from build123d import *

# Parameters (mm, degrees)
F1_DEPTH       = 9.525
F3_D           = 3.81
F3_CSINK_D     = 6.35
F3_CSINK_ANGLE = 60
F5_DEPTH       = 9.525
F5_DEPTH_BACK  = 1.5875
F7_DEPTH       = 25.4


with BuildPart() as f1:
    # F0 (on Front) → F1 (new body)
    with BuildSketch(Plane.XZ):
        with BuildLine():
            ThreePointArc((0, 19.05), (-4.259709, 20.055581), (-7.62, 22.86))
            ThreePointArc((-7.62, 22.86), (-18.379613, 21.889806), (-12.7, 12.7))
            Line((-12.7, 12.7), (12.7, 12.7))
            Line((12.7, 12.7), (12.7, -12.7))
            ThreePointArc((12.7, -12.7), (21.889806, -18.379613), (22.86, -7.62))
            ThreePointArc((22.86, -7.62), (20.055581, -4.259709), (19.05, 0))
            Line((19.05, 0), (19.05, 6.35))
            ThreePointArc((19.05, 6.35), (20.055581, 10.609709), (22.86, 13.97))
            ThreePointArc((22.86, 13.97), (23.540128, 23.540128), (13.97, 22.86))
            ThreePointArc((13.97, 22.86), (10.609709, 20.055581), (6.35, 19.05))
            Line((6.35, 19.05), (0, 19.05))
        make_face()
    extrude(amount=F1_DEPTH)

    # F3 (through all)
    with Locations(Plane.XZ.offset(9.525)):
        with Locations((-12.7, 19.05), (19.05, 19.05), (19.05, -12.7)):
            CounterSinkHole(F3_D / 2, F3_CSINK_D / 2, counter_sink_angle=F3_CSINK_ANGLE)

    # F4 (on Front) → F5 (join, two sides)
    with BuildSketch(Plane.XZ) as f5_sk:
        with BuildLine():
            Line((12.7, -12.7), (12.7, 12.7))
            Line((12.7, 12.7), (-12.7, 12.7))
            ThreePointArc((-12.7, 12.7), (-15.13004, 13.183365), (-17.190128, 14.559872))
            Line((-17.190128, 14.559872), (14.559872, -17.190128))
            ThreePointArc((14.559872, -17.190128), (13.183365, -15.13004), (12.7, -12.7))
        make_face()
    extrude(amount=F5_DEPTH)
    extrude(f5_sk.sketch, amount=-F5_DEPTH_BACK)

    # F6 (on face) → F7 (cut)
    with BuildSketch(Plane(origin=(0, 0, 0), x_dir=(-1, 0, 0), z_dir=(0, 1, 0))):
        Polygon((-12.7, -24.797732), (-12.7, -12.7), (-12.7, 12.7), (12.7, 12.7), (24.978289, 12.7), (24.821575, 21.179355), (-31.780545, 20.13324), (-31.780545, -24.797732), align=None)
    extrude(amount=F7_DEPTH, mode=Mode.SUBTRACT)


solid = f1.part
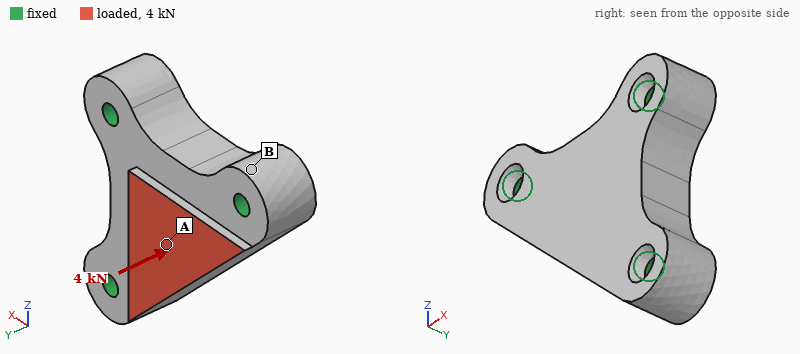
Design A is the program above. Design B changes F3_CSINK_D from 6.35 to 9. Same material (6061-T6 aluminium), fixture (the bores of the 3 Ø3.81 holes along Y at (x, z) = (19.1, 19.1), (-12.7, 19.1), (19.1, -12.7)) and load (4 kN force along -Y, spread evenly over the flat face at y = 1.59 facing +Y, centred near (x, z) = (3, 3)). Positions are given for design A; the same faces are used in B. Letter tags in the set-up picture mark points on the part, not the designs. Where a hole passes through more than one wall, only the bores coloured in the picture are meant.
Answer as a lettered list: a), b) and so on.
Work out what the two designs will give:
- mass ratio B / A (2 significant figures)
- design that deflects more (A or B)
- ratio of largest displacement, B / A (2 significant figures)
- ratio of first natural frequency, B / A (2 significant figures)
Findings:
a) 0.98
b) B
c) 1.3
d) 0.88
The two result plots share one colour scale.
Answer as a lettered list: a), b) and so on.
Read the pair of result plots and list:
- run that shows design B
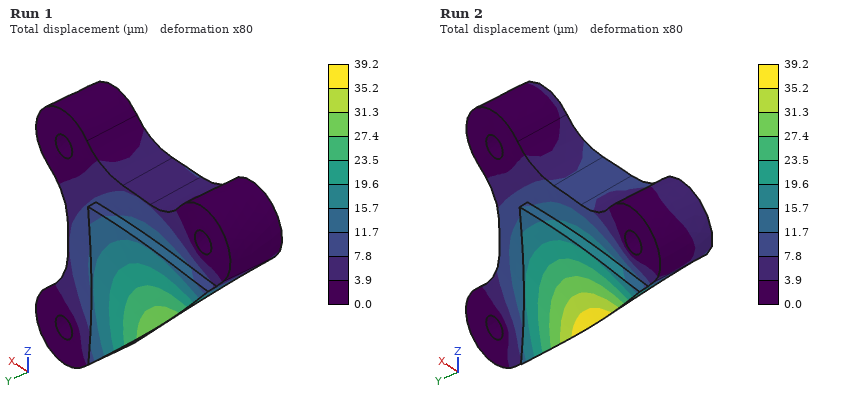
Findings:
a) Run 2
